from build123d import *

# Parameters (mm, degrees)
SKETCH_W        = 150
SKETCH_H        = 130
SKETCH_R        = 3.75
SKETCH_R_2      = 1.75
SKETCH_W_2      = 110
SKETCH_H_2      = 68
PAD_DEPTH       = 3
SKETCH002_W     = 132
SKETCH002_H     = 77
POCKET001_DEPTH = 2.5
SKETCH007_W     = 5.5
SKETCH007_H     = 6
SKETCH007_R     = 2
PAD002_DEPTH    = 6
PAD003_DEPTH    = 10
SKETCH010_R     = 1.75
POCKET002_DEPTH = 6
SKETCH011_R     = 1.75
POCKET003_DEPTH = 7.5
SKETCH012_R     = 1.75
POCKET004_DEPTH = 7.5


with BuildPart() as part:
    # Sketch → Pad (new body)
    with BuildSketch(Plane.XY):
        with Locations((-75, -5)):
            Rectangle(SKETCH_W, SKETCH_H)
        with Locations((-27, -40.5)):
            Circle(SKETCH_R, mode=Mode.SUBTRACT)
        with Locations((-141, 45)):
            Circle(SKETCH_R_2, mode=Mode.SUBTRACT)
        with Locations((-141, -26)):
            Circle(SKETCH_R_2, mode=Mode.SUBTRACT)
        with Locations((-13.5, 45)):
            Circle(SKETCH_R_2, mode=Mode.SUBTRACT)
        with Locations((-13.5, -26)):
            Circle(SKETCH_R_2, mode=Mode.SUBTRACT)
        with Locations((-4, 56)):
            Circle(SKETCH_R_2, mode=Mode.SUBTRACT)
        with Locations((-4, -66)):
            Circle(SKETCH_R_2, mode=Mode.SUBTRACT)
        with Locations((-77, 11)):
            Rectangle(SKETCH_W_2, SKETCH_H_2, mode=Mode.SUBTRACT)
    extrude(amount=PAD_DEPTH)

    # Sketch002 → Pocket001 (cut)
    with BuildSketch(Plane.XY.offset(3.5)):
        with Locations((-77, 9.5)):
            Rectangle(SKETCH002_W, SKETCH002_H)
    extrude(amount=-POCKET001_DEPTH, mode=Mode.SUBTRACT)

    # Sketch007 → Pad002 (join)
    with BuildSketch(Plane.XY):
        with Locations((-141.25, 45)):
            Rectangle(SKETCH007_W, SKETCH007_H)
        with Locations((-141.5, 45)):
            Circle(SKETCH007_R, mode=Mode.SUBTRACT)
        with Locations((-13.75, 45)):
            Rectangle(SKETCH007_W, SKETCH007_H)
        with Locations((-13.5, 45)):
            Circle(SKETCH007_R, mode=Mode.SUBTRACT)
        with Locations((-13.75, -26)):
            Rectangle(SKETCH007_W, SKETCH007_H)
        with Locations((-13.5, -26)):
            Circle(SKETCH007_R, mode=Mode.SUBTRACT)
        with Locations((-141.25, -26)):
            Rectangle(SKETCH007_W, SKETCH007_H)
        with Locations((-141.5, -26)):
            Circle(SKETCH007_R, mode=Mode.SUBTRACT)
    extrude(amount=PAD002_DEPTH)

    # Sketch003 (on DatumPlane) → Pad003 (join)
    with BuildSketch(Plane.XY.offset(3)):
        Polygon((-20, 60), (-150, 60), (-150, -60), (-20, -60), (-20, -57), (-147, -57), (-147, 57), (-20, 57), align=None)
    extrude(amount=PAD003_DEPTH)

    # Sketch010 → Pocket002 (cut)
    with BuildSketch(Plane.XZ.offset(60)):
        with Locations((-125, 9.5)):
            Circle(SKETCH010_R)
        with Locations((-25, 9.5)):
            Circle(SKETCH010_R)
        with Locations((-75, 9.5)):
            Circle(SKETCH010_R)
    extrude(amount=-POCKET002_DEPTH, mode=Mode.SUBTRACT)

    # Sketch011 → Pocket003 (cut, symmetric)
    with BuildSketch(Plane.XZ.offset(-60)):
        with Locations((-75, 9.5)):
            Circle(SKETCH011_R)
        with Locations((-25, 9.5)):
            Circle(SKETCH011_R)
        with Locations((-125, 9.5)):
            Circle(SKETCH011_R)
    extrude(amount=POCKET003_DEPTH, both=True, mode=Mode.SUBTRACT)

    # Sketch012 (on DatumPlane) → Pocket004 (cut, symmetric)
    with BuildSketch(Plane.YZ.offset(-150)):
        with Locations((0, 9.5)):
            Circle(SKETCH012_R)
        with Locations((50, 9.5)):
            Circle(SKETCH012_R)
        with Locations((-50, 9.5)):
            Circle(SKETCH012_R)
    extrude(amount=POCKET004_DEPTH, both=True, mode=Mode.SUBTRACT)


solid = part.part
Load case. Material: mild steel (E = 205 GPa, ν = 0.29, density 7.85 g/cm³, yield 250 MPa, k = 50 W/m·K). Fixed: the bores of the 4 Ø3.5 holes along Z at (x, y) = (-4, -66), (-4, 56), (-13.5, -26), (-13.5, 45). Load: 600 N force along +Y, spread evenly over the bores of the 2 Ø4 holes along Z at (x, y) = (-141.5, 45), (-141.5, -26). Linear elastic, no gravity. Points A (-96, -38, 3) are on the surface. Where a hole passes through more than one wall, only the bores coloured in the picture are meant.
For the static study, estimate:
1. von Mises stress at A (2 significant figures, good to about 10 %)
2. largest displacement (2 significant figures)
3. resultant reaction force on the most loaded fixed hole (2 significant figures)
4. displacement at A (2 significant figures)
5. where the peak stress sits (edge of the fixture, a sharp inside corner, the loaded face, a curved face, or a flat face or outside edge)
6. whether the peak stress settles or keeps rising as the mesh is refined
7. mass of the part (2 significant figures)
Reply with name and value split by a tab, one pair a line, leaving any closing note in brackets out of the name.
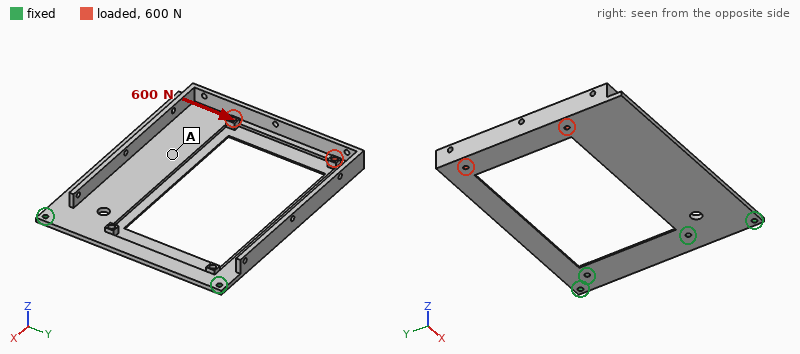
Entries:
von Mises stress at A	17 MPa
largest displacement	0.28 mm
resultant reaction force on the most loaded fixed hole	1.5 kN
displacement at A	0.11 mm
where the peak stress sits	edge of the fixture
whether the peak stress settles or keeps rising as the mesh is refined	keeps rising
mass of the part	330 g
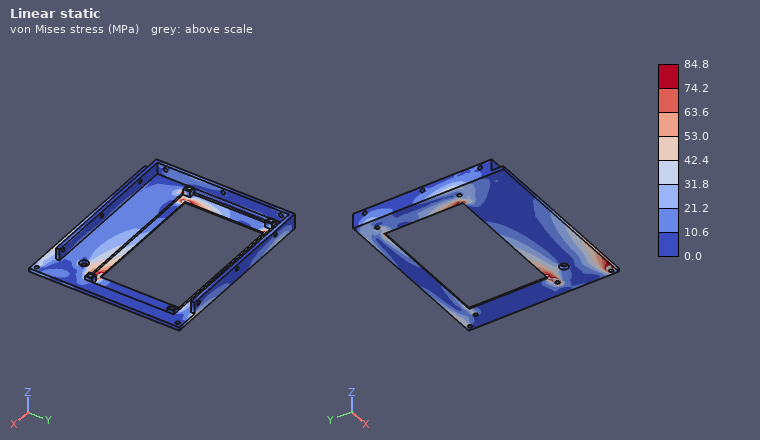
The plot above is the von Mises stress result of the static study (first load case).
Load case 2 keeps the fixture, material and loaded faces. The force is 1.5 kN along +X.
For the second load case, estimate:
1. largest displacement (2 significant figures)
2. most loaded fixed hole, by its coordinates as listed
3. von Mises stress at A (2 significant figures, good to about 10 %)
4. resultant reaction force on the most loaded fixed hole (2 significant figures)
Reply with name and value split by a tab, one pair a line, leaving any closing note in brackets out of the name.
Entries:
largest displacement	0.38 mm
most loaded fixed hole, by its coordinates as listed	(-4, 56)
von Mises stress at A	14 MPa
resultant reaction force on the most loaded fixed hole	780 N
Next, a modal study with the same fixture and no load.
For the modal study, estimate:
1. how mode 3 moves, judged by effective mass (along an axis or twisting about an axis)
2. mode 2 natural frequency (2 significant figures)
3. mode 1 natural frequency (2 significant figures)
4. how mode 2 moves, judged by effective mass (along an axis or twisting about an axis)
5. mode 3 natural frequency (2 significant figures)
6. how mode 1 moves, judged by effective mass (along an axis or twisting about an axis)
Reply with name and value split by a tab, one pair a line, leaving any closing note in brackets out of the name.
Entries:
how mode 3 moves, judged by effective mass	along Y
mode 2 natural frequency	240 Hz
mode 1 natural frequency	120 Hz
how mode 2 moves, judged by effective mass	twisting about X
mode 3 natural frequency	1100 Hz
how mode 1 moves, judged by effective mass	along Z
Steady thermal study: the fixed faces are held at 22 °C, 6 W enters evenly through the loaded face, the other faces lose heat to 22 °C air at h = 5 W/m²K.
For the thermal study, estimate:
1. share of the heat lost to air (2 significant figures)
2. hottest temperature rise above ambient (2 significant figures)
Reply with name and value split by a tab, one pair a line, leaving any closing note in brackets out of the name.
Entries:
share of the heat lost to air	62 %
hottest temperature rise above ambient	62 K
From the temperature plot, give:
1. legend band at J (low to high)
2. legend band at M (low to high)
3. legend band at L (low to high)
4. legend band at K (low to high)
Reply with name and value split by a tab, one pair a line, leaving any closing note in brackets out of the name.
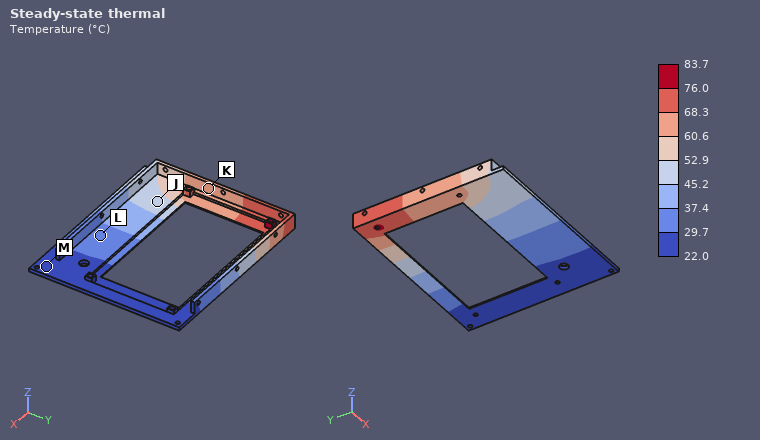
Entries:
legend band at J	45.2 to 52.9 °C
legend band at M	22.0 to 29.7 °C
legend band at L	29.7 to 37.4 °C
legend band at K	60.6 to 68.3 °C
